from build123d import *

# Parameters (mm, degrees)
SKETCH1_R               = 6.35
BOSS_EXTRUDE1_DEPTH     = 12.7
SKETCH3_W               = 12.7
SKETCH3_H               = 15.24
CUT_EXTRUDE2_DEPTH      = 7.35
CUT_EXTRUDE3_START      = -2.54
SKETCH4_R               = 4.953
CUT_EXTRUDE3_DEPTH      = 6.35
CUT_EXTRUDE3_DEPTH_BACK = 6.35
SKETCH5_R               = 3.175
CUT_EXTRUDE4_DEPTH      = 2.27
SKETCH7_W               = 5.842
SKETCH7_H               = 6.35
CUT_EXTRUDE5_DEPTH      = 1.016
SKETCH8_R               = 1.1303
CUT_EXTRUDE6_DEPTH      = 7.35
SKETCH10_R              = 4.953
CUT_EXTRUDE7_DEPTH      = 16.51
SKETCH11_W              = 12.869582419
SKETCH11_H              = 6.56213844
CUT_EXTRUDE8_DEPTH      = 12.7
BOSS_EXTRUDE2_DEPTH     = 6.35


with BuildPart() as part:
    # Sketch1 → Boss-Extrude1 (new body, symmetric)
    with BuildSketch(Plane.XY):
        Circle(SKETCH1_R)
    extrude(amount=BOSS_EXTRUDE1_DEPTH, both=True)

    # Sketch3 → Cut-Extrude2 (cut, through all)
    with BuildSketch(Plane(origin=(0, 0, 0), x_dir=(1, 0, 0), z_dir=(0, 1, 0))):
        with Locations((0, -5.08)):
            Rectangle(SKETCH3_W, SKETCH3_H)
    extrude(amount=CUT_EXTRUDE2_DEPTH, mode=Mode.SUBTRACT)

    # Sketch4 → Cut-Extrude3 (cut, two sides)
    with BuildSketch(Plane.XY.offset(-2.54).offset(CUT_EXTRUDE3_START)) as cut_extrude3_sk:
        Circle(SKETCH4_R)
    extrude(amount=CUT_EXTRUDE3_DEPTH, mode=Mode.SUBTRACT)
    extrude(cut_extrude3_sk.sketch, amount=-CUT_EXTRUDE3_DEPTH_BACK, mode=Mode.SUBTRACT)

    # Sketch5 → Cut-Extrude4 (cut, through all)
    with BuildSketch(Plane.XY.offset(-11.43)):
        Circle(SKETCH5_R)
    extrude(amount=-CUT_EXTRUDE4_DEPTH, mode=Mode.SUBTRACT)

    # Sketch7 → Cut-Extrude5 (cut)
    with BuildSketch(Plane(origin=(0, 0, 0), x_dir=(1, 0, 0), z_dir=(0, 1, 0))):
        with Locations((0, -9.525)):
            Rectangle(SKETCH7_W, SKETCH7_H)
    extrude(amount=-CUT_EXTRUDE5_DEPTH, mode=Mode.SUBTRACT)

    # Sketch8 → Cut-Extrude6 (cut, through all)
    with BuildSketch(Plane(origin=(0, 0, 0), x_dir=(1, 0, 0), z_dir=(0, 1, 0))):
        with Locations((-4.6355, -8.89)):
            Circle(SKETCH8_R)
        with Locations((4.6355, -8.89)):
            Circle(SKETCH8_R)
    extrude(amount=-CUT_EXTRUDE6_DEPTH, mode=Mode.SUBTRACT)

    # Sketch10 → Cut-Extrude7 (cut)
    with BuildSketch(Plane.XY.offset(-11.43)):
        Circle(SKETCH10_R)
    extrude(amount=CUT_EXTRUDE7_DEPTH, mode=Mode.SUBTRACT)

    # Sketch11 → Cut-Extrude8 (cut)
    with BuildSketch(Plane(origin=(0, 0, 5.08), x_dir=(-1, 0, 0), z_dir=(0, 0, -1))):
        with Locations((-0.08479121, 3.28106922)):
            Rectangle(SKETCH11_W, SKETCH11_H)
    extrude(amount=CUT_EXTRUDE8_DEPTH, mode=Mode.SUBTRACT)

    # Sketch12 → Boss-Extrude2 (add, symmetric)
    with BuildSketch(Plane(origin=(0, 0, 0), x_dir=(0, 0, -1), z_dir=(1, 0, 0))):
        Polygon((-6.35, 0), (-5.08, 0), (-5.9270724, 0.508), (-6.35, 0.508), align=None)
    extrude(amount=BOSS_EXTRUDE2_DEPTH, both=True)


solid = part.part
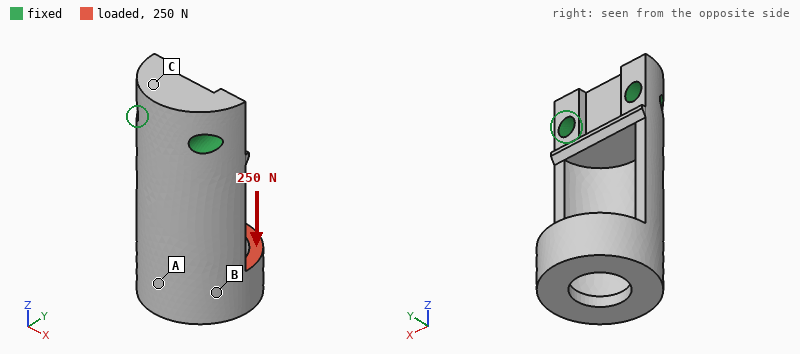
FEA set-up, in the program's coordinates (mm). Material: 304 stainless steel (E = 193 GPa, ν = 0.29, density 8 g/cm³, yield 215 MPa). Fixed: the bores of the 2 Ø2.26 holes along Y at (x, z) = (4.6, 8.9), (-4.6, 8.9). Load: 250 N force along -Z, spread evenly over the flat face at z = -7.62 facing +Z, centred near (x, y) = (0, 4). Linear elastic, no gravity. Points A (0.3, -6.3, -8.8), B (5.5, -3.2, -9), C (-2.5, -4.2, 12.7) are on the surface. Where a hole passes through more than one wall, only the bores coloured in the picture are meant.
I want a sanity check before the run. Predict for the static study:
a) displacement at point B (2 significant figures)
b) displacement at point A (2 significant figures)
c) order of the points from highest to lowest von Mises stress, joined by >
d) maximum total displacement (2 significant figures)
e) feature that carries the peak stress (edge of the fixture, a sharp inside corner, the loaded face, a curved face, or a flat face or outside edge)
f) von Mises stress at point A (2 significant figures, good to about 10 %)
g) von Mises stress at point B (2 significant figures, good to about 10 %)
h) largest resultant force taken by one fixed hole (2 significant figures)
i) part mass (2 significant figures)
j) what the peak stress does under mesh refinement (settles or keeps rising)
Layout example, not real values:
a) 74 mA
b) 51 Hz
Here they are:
a) 17 µm
b) 19 µm
c) B > A > C
d) 44 µm
e) a sharp inside corner
f) 28 MPa
g) 69 MPa
h) 140 N
i) 8.3 g
j) keeps rising
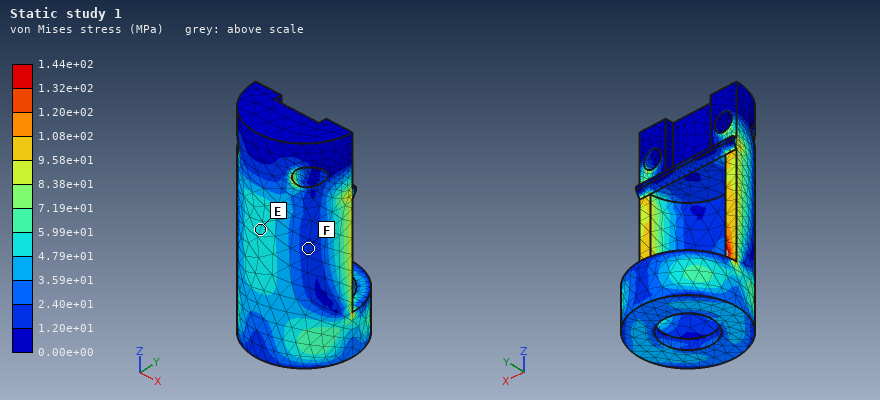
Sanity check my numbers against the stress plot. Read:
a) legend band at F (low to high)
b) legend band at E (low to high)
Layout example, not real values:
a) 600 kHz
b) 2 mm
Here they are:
a) 1.20e+01 to 2.40e+01 MPa
b) 4.79e+01 to 5.99e+01 MPa
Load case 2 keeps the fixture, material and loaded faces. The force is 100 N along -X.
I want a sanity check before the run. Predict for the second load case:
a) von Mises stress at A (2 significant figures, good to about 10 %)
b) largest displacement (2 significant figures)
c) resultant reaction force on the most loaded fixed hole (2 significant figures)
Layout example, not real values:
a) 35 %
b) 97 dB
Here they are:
a) 50 MPa
b) 77 µm
c) 190 N
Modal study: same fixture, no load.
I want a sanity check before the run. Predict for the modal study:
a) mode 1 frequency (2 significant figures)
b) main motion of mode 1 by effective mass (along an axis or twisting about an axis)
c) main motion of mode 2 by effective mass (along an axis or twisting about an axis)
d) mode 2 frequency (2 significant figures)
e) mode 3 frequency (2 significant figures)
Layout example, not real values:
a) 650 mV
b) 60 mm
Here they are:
a) 4800 Hz
b) along X
c) along Y
d) 6700 Hz
e) 19 kHz
